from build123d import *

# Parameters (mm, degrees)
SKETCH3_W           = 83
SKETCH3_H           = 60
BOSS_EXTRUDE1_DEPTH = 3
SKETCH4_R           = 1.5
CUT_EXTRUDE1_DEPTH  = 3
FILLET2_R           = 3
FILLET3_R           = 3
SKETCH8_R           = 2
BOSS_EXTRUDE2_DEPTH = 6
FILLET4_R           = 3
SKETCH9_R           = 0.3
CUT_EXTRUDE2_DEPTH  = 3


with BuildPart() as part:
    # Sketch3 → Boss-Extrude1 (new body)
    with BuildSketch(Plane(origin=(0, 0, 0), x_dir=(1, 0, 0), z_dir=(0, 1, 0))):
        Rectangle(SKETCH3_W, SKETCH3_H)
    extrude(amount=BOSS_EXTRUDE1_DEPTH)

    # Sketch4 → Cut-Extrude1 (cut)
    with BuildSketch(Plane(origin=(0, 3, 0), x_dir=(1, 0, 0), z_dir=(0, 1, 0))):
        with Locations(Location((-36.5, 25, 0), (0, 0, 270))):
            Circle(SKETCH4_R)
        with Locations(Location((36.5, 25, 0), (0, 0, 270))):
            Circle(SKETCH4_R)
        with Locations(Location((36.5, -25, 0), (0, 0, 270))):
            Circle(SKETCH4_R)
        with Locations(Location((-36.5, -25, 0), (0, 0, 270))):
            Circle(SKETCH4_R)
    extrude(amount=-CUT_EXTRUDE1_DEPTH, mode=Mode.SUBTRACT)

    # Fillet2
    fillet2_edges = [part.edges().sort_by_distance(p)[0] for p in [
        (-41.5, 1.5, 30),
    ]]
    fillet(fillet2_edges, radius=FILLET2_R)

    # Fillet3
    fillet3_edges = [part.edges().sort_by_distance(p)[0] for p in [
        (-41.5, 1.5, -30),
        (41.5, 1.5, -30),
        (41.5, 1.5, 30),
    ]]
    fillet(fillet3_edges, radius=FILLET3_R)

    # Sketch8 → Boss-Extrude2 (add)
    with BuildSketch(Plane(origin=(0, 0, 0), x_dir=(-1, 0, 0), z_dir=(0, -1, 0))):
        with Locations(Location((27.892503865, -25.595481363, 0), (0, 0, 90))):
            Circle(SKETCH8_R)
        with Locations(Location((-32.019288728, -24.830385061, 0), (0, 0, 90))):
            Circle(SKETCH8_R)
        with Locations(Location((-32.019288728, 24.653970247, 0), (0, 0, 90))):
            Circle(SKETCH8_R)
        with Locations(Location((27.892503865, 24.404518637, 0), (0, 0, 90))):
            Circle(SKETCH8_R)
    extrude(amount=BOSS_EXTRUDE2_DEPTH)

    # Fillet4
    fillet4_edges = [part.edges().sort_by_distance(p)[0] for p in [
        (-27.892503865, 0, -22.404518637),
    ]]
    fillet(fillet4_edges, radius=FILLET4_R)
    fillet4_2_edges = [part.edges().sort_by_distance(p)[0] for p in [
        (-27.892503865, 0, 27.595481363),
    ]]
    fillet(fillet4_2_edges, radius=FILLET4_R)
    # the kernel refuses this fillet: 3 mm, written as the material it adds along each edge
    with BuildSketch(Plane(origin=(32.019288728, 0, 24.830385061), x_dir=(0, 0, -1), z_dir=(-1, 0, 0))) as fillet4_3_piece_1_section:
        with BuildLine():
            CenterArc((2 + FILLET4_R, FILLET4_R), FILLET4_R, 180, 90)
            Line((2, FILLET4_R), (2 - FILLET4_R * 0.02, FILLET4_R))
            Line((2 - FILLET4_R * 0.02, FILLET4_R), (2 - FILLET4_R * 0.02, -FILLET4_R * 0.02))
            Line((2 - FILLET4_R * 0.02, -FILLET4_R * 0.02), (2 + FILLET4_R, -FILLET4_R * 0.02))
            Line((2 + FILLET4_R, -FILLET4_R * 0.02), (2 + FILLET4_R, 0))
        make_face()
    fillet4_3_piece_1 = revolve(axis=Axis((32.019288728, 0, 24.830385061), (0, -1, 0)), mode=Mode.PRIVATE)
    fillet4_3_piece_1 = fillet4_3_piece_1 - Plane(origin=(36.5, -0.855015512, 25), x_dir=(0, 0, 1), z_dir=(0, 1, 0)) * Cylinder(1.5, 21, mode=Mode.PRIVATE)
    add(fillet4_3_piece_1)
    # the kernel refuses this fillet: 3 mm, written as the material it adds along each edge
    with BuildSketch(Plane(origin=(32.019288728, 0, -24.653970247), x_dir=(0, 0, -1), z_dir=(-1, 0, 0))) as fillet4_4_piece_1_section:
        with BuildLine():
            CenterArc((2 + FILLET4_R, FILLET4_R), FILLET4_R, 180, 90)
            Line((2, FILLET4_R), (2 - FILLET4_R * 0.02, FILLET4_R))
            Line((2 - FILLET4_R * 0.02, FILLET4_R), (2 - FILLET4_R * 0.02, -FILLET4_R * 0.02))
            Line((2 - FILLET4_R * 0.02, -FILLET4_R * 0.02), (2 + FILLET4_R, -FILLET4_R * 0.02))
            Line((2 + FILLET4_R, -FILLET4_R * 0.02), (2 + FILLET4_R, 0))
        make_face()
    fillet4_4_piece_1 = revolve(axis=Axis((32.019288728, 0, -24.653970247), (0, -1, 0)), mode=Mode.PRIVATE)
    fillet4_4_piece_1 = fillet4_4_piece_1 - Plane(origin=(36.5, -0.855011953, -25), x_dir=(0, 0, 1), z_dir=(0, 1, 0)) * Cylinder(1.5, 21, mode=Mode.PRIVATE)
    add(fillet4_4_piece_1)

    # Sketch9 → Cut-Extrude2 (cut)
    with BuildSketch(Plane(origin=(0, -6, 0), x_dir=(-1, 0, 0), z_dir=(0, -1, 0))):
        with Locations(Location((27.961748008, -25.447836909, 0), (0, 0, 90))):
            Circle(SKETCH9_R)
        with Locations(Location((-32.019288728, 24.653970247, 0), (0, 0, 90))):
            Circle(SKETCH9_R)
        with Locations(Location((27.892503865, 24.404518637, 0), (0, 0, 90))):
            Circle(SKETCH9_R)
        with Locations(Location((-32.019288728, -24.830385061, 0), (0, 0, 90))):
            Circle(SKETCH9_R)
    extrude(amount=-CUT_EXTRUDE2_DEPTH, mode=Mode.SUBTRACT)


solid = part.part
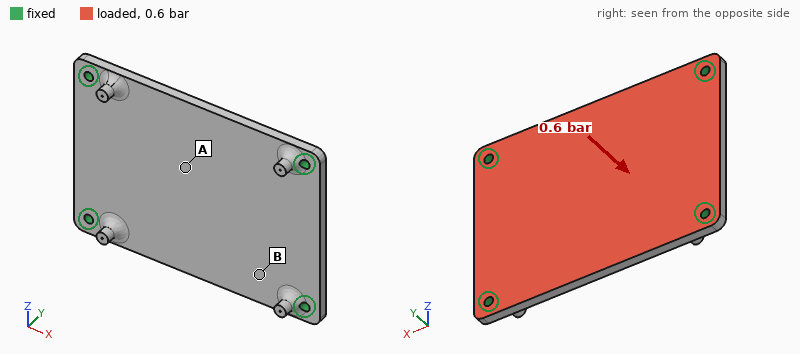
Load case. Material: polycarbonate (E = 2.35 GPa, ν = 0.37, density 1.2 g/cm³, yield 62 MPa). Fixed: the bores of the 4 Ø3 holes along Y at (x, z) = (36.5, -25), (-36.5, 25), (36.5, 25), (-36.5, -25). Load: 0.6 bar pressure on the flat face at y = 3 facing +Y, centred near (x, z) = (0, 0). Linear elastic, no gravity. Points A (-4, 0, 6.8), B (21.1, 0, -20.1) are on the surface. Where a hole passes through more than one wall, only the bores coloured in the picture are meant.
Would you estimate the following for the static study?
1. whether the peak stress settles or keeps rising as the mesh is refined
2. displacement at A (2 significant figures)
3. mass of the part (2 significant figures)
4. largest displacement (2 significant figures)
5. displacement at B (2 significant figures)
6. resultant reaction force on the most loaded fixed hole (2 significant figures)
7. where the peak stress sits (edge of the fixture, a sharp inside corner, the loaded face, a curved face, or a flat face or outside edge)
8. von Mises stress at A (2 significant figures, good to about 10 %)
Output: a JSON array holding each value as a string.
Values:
["keeps rising", "1.2 mm", "18 g", "1.2 mm", "0.52 mm", "80 N", "edge of the fixture", "8.8 MPa"]
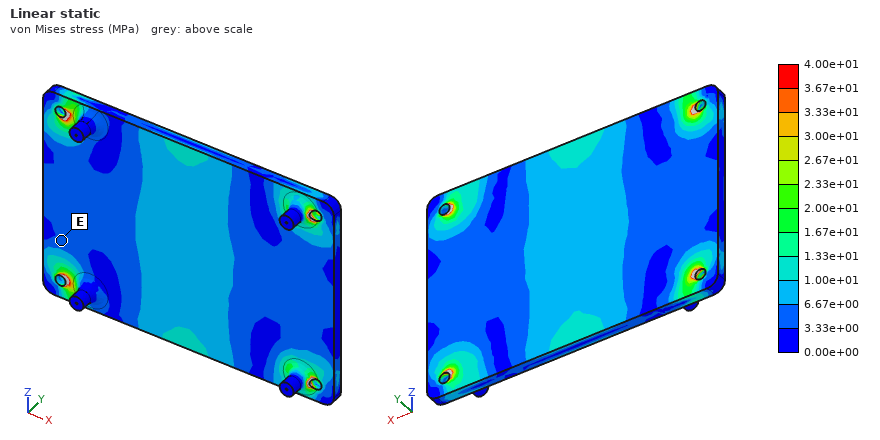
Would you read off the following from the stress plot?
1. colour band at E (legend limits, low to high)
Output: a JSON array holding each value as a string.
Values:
["3.33e+00 to 6.67e+00 MPa"]
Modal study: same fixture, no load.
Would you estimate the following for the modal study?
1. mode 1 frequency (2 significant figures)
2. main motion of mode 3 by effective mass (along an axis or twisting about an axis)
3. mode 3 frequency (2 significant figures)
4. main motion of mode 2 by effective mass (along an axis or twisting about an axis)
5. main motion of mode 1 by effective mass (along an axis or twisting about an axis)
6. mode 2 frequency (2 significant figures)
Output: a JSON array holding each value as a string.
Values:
["700 Hz", "twisting about Z", "1600 Hz", "twisting about X", "along Y", "1100 Hz"]
